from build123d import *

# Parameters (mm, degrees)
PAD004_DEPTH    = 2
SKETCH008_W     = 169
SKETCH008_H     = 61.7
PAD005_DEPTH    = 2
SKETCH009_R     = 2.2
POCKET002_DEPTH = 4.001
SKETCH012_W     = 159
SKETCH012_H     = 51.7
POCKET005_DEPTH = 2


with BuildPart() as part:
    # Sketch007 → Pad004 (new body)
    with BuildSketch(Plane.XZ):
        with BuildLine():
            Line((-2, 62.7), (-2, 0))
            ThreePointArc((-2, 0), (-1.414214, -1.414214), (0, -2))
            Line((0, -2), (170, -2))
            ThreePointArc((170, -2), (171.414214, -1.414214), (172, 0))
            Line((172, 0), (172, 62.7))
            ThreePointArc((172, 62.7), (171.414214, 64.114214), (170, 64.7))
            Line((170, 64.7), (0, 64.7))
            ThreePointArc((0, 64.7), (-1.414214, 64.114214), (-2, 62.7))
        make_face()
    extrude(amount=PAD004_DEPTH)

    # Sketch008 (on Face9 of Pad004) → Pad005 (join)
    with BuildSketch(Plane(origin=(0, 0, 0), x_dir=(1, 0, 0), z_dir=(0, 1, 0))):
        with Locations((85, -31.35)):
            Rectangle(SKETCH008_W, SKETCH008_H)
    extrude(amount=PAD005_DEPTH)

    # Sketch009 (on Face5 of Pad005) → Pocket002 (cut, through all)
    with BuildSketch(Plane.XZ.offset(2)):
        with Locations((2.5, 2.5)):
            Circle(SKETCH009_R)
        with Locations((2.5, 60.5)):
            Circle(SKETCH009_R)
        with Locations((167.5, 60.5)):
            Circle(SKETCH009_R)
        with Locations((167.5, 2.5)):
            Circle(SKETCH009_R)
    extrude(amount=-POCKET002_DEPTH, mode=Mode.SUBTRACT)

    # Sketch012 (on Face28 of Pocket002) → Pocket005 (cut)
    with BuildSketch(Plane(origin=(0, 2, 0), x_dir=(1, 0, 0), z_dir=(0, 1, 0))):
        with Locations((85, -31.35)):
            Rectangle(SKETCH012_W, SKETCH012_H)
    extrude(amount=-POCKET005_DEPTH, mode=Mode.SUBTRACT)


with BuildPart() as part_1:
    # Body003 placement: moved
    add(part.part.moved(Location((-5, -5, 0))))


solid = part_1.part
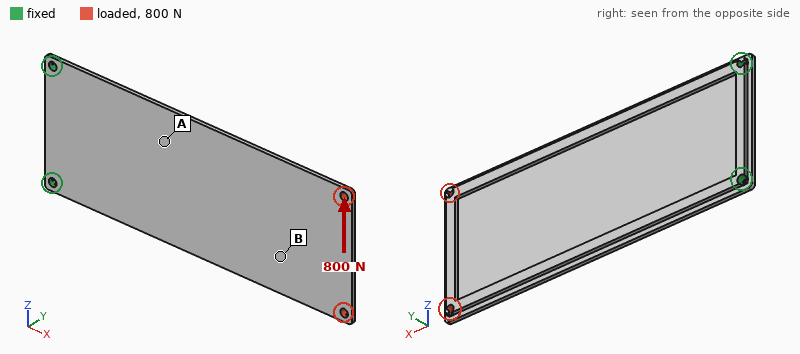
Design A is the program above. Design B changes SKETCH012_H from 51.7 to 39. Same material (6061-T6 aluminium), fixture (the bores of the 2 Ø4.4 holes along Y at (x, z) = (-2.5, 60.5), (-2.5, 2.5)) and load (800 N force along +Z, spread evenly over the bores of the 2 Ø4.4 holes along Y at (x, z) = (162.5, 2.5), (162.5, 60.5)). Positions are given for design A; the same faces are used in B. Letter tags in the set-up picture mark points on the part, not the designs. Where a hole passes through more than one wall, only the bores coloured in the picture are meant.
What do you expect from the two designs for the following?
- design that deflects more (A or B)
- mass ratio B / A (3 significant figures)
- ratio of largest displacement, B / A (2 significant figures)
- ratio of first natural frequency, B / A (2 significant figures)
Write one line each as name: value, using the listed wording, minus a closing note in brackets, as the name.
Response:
design that deflects more: A
mass ratio B / A: 1.15
ratio of largest displacement, B / A: 0.66
ratio of first natural frequency, B / A: 1.2
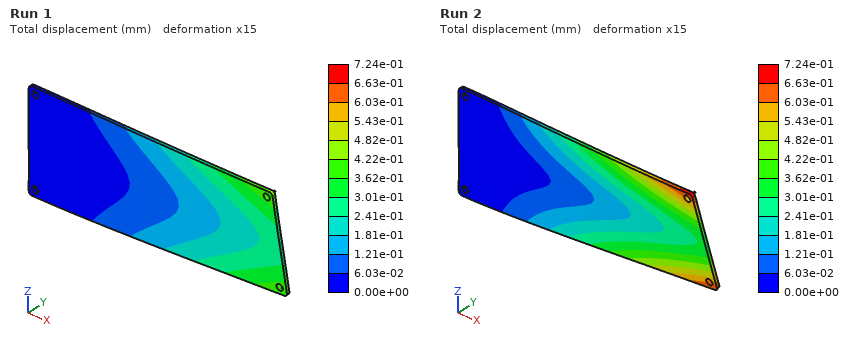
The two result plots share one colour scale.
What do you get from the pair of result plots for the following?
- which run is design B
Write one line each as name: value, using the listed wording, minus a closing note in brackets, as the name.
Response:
which run is design B: Run 1
